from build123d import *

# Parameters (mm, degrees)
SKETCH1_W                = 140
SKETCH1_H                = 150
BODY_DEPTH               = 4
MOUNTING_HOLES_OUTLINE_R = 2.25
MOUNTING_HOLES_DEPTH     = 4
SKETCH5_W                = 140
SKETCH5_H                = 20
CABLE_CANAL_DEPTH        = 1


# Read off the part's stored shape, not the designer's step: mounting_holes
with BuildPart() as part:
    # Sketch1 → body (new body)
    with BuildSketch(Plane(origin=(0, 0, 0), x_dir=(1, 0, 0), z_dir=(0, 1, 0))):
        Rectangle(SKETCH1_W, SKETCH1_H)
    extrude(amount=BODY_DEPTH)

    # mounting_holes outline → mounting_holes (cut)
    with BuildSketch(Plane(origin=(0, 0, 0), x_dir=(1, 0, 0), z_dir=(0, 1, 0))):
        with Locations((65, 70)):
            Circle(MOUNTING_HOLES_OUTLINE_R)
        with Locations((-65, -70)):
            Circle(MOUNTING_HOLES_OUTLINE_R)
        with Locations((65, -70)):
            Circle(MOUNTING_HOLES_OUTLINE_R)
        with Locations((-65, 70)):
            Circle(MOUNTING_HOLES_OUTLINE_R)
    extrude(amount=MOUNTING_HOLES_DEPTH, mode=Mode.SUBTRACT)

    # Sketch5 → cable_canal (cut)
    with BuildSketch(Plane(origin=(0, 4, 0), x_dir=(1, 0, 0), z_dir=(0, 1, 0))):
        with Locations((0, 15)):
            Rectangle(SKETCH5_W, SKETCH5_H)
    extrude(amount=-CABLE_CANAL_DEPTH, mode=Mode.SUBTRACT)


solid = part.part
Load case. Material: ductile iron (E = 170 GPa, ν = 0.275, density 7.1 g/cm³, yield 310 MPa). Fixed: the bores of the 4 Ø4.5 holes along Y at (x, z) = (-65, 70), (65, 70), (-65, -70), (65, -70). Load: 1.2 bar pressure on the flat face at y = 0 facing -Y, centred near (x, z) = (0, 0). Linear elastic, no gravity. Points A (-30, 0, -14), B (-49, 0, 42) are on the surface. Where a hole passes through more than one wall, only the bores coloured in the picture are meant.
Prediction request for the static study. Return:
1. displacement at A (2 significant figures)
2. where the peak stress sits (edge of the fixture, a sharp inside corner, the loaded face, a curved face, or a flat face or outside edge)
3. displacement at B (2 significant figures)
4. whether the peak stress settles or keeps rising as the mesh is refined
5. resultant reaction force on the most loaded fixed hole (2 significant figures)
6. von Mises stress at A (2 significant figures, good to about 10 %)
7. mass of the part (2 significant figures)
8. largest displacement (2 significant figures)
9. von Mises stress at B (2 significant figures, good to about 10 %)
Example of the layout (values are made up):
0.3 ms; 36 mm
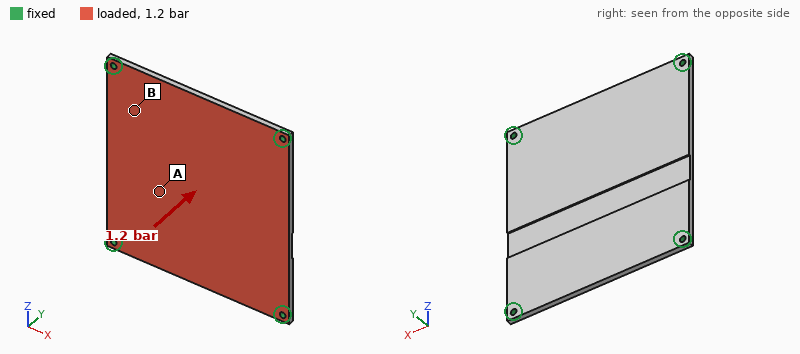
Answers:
0.41 mm; edge of the fixture; 0.19 mm; keeps rising; 770 N; 73 MPa; 570 g; 0.46 mm; 20 MPa
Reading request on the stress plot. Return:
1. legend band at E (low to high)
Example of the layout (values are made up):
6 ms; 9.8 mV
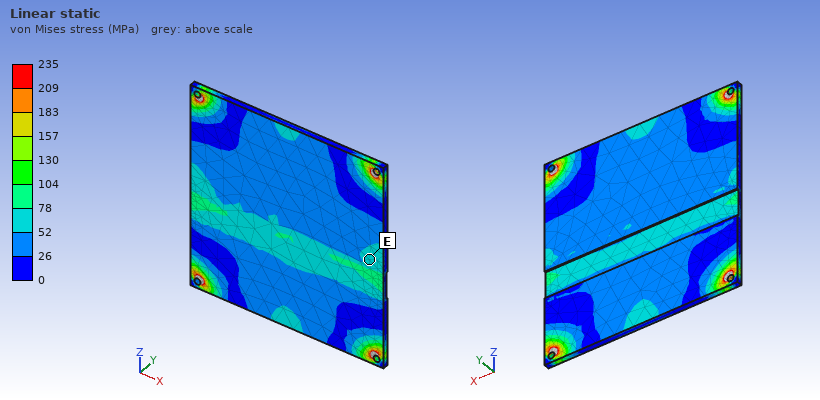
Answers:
52 to 78 MPa
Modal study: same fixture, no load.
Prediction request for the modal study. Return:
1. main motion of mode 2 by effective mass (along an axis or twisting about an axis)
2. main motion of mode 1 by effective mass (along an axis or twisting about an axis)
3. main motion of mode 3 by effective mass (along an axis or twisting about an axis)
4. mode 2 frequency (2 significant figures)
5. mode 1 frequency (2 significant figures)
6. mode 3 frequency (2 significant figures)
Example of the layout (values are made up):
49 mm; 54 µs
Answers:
twisting about Z; along Y; twisting about X; 1100 Hz; 600 Hz; 1200 Hz
